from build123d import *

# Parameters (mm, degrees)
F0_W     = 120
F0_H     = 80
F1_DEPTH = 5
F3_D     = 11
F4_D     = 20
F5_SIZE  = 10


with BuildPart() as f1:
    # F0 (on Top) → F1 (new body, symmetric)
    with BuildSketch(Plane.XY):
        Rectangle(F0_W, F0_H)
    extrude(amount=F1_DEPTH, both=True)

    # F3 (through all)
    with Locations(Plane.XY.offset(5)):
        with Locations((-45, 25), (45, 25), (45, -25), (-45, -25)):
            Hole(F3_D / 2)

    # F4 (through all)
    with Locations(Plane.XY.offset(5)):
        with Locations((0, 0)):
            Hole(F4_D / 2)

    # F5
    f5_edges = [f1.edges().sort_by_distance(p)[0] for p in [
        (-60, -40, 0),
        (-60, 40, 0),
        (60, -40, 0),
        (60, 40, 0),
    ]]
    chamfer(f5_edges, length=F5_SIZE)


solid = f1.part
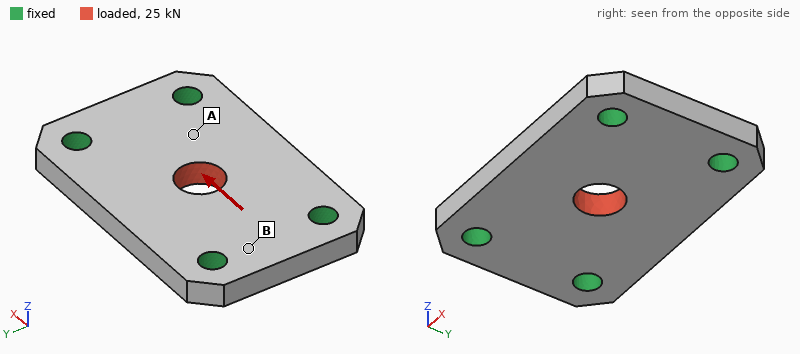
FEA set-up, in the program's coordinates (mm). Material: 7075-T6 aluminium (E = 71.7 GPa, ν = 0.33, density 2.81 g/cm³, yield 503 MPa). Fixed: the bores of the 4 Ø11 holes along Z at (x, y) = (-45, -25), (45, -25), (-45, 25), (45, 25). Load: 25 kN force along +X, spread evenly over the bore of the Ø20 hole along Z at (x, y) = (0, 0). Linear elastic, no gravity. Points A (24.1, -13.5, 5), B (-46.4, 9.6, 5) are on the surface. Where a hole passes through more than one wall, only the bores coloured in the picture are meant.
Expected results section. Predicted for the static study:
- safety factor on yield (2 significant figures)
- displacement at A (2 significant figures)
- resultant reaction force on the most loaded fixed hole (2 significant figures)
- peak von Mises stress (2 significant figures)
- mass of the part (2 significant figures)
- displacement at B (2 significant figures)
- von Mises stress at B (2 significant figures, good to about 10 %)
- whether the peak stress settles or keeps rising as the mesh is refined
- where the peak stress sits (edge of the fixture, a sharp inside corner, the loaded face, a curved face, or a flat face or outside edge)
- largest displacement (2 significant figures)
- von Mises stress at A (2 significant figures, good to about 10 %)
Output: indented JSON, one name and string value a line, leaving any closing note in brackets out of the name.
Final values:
{
  "safety factor on yield": "7.4",
  "displacement at A": "7.7 µm",
  "resultant reaction force on the most loaded fixed hole": "6.6 kN",
  "peak von Mises stress": "68 MPa",
  "mass of the part": "240 g",
  "displacement at B": "4.7 µm",
  "von Mises stress at B": "11 MPa",
  "whether the peak stress settles or keeps rising as the mesh is refined": "settles",
  "where the peak stress sits": "the loaded face",
  "largest displacement": "17 µm",
  "von Mises stress at A": "27 MPa"
}
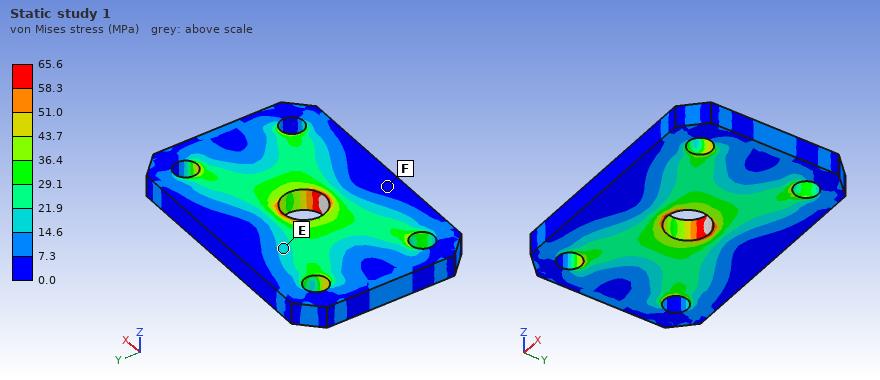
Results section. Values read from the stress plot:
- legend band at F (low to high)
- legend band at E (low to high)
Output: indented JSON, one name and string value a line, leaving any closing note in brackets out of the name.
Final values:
{
  "legend band at F": "0.0 to 7.3 MPa",
  "legend band at E": "14.6 to 21.9 MPa"
}
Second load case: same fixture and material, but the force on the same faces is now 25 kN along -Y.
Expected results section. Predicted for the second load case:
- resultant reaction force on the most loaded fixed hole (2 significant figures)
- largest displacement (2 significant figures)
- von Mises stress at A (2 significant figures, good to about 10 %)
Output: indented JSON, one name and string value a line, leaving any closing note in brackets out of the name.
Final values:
{
  "resultant reaction force on the most loaded fixed hole": "7.6 kN",
  "largest displacement": "33 µm",
  "von Mises stress at A": "35 MPa"
}
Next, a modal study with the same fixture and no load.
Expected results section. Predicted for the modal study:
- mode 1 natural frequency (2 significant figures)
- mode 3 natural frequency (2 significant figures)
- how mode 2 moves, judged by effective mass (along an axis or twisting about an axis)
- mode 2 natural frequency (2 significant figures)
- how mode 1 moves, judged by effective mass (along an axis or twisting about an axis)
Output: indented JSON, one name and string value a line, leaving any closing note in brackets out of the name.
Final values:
{
  "mode 1 natural frequency": "6400 Hz",
  "mode 3 natural frequency": "12 kHz",
  "how mode 2 moves, judged by effective mass": "twisting about X",
  "mode 2 natural frequency": "7800 Hz",
  "how mode 1 moves, judged by effective mass": "along Z"
}
